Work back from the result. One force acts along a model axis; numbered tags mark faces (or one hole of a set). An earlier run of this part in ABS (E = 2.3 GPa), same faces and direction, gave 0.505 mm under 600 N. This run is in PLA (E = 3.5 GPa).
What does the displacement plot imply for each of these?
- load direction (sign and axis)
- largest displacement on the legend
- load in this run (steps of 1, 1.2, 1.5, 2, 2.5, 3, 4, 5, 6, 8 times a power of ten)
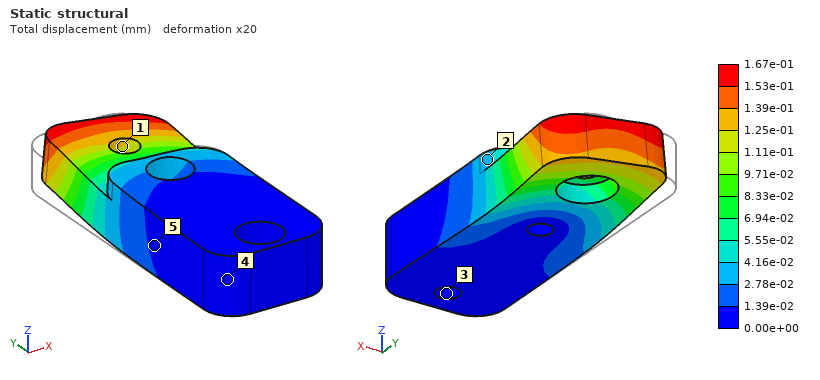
+X
1.67e-01 mm
300 N
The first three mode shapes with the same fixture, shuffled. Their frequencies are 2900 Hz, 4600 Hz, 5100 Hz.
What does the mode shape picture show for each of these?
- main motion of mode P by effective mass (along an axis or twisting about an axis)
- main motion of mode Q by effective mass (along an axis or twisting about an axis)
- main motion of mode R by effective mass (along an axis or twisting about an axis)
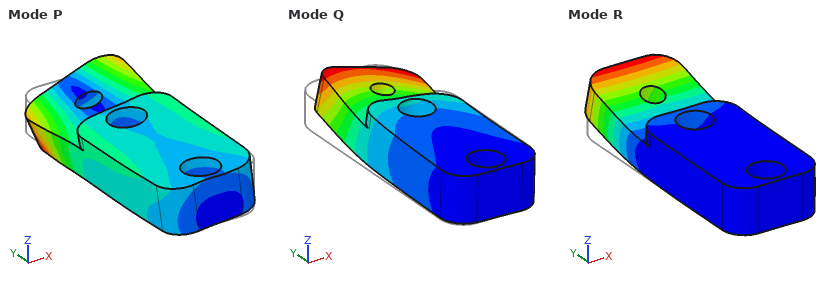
twisting about Y
along X
along Z
